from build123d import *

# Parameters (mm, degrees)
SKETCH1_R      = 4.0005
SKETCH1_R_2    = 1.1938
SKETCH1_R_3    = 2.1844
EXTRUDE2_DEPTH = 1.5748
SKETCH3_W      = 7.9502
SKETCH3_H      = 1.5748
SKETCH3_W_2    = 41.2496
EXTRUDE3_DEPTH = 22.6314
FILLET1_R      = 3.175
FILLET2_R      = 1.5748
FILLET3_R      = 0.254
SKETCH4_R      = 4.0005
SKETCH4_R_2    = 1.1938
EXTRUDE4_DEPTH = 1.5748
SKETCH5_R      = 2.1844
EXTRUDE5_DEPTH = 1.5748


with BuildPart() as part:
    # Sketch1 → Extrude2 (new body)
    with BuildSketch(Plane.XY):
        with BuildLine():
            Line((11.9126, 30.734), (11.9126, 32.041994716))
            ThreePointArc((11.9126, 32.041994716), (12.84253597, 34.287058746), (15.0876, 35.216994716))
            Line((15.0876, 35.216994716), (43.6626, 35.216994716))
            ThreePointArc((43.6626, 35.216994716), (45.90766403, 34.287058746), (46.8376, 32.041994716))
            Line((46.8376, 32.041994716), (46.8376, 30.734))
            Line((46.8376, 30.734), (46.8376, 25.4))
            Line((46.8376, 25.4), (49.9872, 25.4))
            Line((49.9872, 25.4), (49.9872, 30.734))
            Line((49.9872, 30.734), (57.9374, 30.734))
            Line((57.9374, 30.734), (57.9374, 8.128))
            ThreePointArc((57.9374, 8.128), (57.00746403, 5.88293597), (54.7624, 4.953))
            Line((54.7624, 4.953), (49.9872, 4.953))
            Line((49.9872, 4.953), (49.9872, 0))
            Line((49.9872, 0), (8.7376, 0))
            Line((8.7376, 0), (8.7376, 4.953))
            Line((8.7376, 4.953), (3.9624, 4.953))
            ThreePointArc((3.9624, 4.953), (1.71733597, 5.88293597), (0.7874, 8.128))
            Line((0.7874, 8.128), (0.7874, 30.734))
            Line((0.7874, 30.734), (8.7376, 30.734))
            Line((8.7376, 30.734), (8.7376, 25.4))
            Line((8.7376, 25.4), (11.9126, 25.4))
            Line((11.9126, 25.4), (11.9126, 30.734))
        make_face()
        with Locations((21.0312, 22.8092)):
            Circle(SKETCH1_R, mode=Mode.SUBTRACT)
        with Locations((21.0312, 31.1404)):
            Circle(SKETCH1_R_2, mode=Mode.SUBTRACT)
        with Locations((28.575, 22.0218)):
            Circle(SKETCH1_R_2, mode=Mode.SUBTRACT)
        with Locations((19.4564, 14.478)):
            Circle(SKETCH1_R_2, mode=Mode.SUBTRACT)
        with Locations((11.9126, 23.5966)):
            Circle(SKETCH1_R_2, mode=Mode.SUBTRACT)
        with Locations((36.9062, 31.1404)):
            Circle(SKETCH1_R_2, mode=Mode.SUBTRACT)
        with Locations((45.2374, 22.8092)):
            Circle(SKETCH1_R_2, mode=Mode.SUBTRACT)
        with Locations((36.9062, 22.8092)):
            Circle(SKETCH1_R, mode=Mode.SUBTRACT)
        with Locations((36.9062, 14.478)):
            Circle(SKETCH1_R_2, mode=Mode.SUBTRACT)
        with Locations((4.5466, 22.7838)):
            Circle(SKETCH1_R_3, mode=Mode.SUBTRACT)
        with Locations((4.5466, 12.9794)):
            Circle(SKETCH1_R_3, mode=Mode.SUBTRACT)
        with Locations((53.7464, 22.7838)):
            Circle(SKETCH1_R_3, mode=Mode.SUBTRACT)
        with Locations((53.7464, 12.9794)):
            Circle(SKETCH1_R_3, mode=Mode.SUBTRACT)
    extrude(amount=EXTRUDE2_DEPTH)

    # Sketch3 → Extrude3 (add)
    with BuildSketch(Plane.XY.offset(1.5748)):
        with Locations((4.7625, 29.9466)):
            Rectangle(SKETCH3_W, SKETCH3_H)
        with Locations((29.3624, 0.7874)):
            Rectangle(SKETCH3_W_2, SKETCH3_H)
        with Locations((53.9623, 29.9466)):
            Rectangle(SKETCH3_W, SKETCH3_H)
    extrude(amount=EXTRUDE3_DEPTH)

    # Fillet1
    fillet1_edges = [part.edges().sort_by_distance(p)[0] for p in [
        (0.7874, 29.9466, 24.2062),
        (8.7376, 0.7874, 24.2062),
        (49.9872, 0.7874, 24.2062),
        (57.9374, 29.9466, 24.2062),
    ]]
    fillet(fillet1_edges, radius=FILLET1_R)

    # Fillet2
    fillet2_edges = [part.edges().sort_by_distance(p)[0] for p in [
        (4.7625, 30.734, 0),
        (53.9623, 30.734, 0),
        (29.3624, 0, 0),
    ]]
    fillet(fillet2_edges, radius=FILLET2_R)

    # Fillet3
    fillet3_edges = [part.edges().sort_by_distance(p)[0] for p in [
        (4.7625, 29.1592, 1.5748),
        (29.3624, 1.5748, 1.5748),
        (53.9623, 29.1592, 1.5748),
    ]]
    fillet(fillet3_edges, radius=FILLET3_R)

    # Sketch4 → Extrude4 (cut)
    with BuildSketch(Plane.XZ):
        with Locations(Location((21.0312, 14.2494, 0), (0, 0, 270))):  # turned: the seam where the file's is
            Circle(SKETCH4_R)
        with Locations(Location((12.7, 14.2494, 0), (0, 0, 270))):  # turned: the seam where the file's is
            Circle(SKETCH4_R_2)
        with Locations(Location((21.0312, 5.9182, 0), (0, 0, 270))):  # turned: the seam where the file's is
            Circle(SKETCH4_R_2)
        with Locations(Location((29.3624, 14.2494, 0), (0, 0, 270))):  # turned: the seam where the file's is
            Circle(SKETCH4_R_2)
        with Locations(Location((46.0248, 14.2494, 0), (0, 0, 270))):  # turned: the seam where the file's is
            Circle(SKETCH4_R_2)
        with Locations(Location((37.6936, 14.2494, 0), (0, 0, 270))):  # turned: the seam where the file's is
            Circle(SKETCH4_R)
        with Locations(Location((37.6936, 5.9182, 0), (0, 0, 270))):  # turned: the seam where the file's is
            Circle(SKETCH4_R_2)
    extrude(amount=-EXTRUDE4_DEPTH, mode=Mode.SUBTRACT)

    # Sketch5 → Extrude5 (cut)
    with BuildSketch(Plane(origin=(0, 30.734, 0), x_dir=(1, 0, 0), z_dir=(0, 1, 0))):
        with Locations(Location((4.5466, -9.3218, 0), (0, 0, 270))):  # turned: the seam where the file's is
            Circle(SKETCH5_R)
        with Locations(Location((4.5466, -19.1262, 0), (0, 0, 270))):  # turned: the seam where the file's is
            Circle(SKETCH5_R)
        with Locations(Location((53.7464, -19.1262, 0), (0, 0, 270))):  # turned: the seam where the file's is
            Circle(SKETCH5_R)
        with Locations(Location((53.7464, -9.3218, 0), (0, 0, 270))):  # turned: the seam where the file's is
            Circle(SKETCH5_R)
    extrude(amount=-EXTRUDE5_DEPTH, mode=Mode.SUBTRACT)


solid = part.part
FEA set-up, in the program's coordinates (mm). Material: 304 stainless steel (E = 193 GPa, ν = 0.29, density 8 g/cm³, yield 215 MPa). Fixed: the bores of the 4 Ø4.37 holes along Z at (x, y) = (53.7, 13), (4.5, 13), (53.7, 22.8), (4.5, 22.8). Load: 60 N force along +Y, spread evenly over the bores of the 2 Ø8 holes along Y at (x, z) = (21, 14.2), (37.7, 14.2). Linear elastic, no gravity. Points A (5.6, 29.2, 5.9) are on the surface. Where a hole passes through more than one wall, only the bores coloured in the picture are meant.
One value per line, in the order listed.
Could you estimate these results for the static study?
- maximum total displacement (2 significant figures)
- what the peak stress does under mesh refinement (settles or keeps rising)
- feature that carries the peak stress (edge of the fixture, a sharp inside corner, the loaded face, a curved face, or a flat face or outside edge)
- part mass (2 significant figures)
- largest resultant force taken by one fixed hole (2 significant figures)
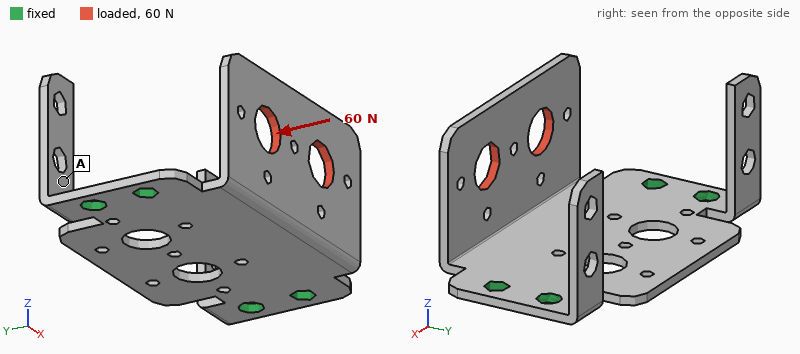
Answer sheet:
0.13 mm
keeps rising
a sharp inside corner
34 g
27 N
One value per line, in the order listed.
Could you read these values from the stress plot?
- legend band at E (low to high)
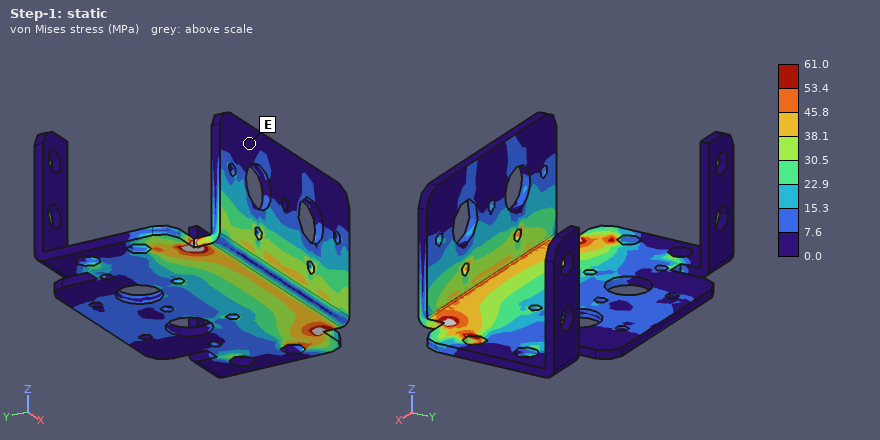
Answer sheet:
0.0 to 7.6 MPa
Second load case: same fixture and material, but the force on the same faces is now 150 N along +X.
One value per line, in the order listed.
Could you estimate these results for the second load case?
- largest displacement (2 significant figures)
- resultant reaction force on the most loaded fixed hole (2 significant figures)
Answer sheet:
41 µm
88 N
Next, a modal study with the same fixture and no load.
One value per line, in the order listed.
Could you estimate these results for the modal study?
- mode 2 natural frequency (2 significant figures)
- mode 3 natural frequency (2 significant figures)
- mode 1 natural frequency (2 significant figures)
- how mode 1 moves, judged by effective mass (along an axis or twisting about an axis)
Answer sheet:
1800 Hz
1800 Hz
1300 Hz
along Y
